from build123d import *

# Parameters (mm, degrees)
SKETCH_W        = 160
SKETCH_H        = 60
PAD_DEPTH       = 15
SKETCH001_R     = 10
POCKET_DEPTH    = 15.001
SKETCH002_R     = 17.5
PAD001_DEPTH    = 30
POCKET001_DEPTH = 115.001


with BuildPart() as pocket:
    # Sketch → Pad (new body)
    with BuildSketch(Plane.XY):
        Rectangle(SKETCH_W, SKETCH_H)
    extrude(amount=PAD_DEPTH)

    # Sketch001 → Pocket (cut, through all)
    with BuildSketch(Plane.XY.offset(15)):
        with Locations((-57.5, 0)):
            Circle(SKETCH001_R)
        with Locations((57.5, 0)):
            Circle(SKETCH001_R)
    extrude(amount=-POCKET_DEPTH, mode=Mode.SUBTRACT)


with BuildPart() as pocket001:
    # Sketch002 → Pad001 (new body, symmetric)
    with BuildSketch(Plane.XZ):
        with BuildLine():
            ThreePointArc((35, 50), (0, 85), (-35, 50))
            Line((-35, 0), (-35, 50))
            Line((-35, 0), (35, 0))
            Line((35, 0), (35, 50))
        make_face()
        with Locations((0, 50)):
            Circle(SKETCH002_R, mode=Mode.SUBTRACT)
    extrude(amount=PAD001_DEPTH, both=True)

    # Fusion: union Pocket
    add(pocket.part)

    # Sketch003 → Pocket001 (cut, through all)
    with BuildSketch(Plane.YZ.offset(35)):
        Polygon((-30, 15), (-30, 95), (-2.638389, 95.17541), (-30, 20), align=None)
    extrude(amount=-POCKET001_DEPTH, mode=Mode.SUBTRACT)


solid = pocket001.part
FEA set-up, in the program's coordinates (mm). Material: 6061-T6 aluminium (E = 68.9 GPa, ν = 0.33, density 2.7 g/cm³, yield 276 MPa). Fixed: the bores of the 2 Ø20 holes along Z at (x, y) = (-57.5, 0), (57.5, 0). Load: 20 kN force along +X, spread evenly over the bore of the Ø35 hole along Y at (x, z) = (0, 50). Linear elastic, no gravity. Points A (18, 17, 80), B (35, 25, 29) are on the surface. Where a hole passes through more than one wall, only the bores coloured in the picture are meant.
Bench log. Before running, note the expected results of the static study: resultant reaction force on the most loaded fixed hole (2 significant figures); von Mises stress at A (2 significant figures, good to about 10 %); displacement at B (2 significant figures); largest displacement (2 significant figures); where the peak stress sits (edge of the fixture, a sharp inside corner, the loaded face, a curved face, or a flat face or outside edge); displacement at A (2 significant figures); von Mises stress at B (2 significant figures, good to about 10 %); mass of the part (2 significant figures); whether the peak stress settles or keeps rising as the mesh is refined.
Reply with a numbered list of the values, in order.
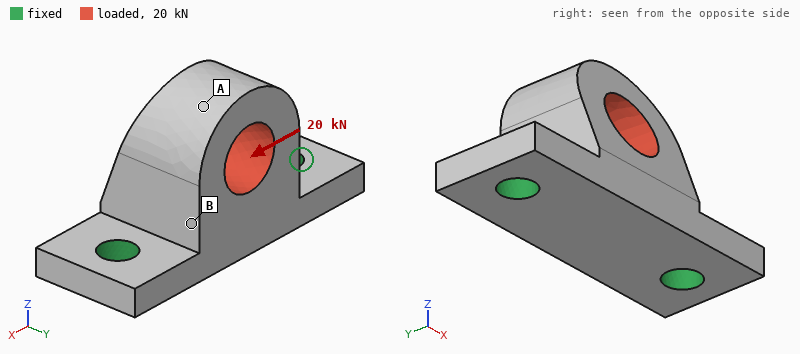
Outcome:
1. 14 kN
2. 8.9 MPa
3. 30 µm
4. 74 µm
5. edge of the fixture
6. 72 µm
7. 18 MPa
8. 830 g
9. keeps rising
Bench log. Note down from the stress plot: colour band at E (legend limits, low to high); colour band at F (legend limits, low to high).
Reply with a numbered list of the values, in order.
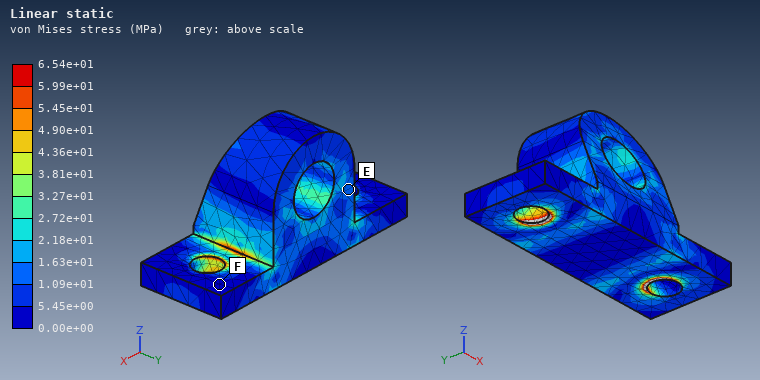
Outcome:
1. 1.09e+01 to 1.63e+01 MPa
2. 0.00e+00 to 5.45e+00 MPa
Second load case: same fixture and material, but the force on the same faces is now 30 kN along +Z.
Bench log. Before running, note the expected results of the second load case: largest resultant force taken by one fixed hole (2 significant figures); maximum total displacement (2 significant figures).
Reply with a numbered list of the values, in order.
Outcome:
1. 16 kN
2. 97 µm
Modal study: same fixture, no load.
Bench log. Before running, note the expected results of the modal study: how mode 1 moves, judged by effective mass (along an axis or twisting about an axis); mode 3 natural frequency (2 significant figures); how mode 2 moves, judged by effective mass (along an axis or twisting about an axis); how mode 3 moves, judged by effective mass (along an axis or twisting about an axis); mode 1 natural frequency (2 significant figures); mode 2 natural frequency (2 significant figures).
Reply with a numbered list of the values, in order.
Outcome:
1. along Y
2. 5200 Hz
3. along X
4. along Z
5. 2200 Hz
6. 4800 Hz
